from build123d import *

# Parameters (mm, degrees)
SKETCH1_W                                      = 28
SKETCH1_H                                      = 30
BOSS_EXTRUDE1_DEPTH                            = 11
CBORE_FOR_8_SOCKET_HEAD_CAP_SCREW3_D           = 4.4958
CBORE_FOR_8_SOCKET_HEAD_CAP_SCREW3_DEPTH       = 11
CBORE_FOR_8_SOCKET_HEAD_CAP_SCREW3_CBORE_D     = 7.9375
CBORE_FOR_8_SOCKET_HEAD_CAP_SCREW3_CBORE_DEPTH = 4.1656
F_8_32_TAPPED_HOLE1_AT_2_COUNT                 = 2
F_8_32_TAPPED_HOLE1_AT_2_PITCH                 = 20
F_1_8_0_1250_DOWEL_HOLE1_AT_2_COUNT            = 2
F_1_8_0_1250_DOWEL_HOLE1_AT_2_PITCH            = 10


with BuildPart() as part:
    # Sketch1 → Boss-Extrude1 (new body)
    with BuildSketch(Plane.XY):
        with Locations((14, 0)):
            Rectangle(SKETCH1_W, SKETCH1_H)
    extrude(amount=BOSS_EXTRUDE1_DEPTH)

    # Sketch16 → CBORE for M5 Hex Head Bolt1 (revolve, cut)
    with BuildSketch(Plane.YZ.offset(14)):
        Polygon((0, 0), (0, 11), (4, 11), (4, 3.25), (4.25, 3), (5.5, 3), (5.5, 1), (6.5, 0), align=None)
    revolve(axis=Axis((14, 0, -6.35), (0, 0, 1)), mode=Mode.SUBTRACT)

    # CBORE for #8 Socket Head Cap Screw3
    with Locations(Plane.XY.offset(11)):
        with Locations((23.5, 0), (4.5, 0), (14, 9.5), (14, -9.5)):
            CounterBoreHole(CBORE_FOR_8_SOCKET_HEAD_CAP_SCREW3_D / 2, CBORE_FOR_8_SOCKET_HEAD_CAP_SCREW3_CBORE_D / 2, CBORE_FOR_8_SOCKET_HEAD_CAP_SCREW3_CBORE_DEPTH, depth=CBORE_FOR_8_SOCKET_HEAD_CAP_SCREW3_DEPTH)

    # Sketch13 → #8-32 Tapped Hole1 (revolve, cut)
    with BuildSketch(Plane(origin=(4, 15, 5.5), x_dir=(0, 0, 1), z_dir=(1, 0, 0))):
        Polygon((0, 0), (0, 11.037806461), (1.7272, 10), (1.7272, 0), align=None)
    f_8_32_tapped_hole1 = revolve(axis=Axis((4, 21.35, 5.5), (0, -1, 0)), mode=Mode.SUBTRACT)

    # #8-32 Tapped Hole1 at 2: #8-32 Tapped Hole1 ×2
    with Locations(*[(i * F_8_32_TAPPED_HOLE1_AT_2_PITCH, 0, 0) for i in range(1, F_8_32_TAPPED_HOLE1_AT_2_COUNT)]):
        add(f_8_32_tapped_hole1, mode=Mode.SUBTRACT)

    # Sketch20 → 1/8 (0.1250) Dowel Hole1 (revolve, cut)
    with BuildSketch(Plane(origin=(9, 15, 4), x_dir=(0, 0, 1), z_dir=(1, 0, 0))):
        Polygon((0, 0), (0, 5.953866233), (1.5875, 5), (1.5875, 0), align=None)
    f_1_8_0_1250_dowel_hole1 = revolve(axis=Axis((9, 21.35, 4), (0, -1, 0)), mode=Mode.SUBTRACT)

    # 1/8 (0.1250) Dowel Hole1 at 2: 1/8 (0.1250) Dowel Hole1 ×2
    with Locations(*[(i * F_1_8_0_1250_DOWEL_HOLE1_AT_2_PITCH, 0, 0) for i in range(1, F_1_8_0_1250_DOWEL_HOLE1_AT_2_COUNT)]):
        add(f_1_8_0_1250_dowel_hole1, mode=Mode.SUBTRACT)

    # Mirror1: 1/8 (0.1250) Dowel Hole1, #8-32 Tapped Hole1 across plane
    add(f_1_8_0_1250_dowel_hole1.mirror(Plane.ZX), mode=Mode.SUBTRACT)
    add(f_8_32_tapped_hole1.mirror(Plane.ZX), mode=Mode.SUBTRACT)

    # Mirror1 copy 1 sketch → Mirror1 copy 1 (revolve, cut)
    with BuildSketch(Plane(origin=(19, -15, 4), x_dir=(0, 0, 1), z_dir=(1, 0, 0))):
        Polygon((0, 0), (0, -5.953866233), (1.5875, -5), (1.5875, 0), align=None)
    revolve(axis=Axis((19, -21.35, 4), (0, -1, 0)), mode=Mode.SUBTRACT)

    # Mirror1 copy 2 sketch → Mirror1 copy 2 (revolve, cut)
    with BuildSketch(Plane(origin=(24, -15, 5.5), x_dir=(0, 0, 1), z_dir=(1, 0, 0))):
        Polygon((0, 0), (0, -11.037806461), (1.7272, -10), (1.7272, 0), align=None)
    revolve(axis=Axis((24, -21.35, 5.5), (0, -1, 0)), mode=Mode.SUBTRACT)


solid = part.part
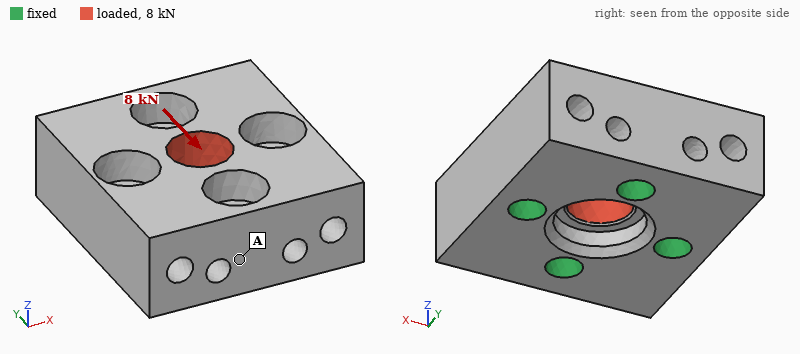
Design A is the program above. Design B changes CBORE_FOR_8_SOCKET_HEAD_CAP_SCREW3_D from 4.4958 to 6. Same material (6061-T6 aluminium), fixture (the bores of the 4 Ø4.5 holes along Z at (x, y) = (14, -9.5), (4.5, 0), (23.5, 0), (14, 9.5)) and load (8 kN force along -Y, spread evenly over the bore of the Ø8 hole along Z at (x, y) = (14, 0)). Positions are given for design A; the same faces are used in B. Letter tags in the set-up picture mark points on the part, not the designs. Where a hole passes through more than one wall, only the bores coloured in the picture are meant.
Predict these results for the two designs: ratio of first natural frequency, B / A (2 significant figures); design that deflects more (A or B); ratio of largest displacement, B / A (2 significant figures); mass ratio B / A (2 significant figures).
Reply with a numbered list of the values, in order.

1. 1.1
2. A
3. 0.92
4. 0.95
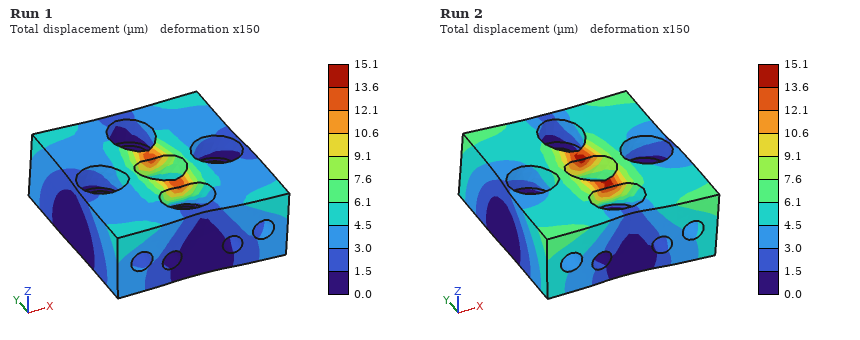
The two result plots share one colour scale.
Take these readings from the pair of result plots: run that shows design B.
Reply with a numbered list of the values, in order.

1. Run 1
